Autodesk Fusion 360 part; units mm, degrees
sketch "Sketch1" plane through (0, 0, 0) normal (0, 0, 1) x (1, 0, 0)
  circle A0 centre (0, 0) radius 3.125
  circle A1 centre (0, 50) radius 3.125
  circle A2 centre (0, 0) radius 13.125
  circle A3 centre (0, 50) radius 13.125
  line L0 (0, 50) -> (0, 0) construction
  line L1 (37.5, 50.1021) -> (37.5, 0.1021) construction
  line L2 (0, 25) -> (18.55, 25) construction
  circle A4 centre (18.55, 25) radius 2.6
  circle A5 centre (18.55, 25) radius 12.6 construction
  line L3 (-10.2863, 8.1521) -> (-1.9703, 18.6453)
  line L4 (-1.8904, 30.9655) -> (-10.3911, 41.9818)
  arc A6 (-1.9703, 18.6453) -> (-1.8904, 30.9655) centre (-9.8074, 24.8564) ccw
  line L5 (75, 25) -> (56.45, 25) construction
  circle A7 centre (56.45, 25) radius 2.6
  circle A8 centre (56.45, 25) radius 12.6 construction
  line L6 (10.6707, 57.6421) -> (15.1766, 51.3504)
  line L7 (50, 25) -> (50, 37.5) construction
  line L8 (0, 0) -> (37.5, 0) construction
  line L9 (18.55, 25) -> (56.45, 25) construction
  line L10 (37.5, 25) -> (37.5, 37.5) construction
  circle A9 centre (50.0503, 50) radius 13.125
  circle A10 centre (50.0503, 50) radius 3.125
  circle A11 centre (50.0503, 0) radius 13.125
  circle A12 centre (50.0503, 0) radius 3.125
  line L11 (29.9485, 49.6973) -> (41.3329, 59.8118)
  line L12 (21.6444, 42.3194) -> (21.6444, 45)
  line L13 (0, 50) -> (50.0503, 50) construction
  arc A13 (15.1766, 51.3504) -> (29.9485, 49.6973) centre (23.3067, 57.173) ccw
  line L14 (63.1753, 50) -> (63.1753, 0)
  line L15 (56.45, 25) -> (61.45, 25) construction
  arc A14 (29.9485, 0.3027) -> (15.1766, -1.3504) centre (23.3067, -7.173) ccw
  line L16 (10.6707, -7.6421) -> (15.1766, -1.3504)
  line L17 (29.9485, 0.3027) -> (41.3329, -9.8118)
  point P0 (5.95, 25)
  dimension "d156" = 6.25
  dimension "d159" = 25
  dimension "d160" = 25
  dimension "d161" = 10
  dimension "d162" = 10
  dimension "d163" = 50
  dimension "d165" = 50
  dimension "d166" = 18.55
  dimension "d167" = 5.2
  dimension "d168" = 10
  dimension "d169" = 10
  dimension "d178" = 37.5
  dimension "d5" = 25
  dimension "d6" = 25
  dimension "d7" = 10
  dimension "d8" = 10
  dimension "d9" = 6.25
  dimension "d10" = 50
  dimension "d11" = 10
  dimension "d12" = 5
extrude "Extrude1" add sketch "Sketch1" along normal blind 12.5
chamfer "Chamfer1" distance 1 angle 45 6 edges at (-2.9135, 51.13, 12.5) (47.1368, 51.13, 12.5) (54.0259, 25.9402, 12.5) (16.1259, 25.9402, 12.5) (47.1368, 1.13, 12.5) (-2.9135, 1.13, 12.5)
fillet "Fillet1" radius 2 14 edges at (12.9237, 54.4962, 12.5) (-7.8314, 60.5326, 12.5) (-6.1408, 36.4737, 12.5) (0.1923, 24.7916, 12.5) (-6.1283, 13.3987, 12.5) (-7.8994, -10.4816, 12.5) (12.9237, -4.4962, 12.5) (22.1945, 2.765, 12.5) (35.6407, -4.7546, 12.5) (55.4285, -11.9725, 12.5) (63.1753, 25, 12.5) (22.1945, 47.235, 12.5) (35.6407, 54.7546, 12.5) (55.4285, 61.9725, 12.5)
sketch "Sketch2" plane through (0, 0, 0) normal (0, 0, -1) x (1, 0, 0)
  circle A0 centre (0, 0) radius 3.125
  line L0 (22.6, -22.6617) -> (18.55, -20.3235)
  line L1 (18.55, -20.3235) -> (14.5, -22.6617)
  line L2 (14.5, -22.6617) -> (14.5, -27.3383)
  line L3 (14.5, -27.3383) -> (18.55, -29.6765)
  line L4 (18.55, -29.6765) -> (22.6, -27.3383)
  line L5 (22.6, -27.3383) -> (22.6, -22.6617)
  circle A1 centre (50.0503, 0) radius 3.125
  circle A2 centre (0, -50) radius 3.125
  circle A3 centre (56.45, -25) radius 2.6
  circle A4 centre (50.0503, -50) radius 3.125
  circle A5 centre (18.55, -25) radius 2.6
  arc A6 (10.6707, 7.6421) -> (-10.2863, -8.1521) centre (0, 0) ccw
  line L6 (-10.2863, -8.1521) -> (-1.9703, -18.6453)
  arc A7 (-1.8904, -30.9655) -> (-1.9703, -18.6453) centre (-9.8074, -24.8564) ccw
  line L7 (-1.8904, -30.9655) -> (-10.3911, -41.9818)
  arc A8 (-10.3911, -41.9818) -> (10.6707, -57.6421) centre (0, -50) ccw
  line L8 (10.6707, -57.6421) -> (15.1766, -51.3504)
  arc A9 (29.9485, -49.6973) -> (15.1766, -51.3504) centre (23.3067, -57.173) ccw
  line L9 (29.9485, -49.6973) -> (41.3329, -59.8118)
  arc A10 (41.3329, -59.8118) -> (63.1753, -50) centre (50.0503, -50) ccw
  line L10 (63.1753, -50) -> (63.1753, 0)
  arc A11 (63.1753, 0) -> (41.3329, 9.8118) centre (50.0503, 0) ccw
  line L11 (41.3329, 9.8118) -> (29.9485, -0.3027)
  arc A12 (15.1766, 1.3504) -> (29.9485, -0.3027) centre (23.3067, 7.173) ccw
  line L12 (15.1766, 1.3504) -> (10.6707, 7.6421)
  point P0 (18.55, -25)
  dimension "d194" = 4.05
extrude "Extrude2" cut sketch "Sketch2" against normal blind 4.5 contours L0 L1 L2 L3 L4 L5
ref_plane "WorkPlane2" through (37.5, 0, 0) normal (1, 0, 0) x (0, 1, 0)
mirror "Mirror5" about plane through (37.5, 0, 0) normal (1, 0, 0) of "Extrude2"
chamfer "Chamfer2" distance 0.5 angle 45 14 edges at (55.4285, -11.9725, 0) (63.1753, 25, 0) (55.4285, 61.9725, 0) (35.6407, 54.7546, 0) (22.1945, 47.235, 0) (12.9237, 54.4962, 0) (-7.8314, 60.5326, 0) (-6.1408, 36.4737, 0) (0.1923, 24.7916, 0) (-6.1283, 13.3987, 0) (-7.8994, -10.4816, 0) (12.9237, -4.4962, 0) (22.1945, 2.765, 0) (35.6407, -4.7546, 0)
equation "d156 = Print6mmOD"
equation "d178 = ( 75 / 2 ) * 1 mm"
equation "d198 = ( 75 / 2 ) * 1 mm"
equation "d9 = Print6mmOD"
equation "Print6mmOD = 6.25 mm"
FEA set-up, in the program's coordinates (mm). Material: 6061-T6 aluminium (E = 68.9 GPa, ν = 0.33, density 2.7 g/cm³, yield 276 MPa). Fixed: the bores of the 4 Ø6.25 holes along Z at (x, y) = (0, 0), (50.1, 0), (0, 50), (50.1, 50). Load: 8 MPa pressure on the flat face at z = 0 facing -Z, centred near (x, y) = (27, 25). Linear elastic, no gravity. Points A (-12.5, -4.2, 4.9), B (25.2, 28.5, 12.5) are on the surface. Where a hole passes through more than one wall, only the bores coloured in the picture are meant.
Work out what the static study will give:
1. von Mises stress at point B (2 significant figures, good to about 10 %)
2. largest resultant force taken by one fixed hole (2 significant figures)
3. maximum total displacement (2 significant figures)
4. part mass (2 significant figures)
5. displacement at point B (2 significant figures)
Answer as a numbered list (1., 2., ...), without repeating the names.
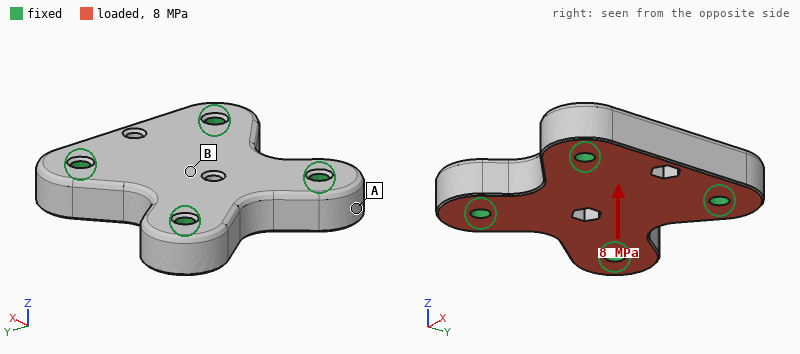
1. 40 MPa
2. 9.1 kN
3. 41 µm
4. 150 g
5. 39 µm
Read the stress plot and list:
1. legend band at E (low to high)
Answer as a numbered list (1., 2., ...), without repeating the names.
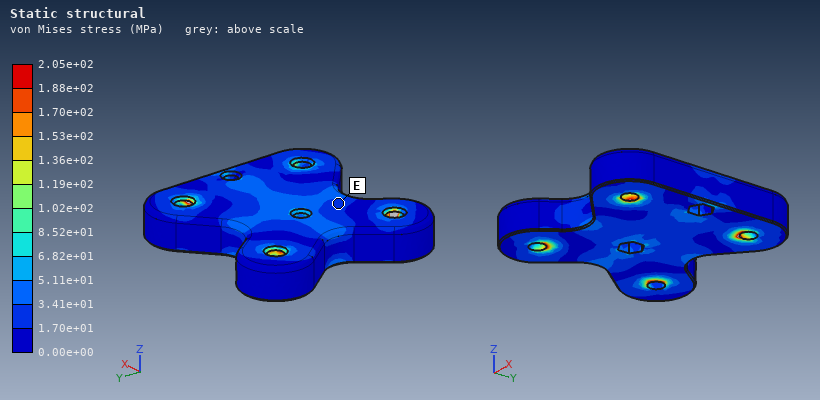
1. 1.70e+01 to 3.41e+01 MPa
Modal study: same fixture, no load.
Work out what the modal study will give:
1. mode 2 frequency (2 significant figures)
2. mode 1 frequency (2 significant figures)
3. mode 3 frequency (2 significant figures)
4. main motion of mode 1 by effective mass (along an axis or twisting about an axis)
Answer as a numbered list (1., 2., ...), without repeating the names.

1. 20 kHz
2. 14 kHz
3. 25 kHz
4. along Z
